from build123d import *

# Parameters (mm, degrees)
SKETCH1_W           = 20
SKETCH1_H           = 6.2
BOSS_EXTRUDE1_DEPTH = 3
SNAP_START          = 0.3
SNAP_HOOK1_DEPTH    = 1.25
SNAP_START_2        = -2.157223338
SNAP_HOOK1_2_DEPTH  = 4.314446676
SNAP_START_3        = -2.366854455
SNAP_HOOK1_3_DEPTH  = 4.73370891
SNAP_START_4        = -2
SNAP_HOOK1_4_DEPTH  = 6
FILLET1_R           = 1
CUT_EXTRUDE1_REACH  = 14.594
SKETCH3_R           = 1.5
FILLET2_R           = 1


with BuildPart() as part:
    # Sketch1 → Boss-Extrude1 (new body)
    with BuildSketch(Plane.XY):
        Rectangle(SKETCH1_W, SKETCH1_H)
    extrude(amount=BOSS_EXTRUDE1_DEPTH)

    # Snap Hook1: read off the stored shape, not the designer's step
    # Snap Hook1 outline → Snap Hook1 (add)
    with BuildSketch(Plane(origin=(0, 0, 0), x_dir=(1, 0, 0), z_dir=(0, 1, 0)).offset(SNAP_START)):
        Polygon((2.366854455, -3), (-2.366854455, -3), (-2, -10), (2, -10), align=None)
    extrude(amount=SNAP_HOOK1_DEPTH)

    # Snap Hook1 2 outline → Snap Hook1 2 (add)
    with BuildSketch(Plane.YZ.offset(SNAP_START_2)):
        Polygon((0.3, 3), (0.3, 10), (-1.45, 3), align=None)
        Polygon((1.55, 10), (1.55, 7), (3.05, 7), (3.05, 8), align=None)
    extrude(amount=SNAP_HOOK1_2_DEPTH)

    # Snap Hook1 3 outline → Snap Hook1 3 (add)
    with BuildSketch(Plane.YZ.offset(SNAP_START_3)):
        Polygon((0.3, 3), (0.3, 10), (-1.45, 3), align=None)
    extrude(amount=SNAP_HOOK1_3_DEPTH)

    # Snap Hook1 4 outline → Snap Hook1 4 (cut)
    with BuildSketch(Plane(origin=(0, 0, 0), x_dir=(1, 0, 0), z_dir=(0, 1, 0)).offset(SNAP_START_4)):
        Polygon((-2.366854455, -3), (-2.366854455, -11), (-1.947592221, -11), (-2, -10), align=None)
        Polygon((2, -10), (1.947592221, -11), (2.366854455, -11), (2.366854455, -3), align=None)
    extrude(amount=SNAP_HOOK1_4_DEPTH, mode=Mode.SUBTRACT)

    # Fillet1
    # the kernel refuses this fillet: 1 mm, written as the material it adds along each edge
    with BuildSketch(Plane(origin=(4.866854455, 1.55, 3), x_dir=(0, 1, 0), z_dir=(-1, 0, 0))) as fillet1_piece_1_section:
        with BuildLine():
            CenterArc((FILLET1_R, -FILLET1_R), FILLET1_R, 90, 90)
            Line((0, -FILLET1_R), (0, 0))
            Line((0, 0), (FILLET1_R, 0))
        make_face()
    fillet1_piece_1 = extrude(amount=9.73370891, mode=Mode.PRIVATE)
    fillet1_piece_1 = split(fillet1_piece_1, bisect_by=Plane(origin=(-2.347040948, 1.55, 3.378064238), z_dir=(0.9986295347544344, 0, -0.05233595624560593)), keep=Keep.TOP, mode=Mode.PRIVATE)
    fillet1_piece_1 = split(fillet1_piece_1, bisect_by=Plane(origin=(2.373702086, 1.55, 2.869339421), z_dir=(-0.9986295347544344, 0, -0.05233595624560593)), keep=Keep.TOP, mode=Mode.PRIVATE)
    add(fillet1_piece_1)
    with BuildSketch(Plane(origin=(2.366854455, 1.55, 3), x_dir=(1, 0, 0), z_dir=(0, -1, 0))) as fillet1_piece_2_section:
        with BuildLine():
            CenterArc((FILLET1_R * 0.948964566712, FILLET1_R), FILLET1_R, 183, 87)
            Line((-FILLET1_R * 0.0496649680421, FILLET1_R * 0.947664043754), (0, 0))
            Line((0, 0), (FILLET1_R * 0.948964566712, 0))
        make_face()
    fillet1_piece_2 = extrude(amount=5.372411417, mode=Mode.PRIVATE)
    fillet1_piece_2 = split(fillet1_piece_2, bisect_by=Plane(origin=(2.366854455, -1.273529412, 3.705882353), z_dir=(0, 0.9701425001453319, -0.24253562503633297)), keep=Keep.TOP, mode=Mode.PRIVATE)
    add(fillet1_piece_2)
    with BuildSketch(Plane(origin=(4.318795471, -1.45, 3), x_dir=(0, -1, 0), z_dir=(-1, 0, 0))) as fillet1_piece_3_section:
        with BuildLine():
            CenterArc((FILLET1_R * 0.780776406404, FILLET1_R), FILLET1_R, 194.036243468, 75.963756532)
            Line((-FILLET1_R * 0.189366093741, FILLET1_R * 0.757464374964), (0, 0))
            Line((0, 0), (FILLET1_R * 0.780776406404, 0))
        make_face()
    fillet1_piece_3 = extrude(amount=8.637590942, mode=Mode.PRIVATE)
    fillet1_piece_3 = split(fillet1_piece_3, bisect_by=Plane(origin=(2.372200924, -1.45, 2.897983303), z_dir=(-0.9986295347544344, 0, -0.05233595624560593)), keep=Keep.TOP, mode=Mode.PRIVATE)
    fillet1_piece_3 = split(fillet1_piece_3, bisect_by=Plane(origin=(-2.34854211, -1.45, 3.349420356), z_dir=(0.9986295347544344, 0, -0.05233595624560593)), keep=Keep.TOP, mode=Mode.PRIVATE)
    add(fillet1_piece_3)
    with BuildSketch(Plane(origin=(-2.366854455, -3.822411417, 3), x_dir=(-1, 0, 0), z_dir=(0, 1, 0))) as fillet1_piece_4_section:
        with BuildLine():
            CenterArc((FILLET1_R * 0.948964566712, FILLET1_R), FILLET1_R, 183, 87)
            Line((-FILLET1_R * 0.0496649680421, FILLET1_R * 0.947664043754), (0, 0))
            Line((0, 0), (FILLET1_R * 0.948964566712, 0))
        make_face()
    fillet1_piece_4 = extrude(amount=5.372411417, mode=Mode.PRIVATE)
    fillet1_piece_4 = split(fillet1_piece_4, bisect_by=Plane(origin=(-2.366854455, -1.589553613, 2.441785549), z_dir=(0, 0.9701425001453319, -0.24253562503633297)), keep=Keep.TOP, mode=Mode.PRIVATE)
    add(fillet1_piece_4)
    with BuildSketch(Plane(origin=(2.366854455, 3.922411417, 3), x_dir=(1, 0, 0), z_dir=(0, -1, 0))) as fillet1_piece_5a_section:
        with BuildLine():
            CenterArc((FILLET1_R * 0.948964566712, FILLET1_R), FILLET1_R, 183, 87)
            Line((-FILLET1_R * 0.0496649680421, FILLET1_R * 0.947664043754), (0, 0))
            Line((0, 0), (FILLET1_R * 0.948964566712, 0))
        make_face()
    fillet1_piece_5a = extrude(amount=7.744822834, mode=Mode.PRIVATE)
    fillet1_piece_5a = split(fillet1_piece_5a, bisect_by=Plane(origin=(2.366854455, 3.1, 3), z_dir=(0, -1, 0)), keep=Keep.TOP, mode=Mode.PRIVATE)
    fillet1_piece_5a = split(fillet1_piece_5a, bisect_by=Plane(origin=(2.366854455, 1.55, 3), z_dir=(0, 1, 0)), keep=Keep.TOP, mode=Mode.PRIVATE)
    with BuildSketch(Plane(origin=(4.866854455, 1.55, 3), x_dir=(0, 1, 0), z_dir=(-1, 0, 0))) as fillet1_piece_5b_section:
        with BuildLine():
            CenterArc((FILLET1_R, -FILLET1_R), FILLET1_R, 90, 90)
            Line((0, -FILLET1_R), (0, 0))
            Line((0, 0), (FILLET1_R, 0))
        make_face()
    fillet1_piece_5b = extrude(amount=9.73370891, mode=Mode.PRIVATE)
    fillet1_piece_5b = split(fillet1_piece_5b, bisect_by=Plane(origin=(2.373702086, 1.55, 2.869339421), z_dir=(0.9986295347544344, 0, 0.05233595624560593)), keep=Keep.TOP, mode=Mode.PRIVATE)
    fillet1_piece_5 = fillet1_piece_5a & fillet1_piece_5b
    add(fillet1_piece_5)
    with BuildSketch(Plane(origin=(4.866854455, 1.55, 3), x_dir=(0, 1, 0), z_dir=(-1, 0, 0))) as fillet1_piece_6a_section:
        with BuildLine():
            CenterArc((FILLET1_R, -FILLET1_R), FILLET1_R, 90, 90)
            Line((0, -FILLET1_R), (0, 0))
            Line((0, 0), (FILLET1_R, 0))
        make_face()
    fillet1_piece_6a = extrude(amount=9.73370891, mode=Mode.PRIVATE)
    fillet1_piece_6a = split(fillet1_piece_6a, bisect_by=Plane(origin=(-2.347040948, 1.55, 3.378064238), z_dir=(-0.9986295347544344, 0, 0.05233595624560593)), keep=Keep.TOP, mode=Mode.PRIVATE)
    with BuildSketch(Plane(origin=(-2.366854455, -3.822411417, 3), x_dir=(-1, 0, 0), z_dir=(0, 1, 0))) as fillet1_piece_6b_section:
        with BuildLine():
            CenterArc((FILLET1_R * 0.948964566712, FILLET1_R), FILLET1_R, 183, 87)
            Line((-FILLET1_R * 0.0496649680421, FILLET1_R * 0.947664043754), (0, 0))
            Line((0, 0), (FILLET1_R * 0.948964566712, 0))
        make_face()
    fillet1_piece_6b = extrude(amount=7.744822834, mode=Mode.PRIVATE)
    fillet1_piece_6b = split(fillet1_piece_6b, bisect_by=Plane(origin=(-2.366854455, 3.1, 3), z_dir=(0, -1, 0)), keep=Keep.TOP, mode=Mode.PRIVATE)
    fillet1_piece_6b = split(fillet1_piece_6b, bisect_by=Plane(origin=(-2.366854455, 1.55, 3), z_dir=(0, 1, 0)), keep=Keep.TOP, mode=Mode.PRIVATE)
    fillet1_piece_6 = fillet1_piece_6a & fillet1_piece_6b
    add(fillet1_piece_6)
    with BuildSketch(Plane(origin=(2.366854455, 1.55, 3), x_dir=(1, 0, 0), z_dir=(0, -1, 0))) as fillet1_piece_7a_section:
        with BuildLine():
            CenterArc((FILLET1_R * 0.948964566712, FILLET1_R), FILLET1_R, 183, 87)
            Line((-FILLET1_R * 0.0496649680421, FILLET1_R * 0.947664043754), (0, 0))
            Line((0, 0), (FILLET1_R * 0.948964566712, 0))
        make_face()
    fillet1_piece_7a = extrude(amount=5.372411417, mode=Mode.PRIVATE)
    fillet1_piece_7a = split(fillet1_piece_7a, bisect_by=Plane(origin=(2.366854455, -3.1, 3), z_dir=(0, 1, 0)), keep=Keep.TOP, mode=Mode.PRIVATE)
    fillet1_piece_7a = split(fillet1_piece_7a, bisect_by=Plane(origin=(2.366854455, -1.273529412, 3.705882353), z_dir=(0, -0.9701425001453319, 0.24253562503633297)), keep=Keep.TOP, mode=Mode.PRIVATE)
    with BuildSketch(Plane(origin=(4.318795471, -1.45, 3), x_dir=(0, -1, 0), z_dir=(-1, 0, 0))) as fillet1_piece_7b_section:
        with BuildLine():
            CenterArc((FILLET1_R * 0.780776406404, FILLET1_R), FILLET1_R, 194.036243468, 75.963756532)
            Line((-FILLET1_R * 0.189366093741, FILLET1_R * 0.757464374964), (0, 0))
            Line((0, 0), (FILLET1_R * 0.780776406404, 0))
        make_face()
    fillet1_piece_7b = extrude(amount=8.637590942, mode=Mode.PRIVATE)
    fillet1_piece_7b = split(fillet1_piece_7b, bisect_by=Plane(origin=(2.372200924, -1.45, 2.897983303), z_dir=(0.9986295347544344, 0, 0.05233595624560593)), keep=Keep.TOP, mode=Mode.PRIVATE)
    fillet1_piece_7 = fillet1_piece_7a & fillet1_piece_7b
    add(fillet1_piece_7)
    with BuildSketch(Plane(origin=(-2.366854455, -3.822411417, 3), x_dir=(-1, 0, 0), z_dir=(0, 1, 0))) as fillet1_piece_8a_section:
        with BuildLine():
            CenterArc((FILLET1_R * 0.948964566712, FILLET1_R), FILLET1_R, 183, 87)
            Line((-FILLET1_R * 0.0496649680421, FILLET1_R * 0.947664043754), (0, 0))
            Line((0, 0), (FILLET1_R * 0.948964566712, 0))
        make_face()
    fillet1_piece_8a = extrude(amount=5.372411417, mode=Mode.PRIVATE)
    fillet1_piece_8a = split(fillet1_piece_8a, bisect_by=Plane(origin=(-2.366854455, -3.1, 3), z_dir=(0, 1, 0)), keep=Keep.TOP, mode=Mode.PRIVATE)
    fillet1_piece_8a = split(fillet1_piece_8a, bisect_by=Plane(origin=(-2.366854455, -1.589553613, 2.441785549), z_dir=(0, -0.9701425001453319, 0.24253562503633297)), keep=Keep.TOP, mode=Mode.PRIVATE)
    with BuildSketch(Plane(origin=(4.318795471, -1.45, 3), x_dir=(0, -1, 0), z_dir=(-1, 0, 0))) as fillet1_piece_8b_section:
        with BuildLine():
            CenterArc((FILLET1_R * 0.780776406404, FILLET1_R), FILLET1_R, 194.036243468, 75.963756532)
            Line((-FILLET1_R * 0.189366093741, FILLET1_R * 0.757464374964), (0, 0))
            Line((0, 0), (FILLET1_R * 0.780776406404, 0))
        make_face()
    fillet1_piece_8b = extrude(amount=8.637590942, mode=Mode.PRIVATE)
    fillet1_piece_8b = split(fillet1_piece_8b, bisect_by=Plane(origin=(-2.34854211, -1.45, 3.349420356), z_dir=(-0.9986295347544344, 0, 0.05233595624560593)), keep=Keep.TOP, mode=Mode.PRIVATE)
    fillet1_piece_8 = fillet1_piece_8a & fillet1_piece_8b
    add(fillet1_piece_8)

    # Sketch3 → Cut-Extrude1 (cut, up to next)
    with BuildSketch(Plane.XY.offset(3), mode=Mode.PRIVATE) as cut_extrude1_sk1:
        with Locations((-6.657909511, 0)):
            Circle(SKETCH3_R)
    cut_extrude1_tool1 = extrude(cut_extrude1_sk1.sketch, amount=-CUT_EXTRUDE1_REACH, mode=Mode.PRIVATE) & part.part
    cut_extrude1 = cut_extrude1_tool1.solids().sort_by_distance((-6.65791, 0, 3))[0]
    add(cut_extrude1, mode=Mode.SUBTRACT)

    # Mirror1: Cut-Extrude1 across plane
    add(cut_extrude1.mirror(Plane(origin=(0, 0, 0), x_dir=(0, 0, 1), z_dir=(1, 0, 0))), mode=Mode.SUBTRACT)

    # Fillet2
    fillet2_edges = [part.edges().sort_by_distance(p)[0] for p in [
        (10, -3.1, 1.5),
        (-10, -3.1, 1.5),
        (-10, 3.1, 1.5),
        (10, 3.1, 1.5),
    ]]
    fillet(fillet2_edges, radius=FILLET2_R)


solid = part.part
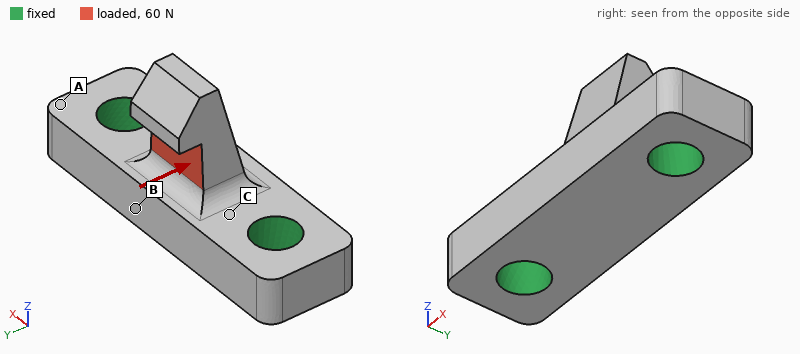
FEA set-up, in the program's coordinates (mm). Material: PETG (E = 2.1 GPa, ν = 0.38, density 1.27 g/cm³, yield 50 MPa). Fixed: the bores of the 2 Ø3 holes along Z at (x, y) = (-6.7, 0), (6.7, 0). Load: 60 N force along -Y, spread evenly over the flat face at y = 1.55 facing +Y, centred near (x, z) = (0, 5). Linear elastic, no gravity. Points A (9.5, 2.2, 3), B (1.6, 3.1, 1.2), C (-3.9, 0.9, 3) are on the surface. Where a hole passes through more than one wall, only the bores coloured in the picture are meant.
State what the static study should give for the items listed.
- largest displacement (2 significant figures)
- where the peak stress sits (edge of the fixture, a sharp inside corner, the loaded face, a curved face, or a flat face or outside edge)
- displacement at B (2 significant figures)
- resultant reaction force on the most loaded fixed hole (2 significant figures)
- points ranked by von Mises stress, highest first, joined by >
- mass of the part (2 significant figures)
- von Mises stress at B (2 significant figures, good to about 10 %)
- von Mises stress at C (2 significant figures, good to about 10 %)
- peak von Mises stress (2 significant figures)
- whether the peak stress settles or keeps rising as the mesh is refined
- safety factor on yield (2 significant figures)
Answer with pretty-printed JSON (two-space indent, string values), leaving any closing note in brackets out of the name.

{
  "largest displacement": "0.22 mm",
  "where the peak stress sits": "a curved face",
  "displacement at B": "0.039 mm",
  "resultant reaction force on the most loaded fixed hole": "30 N",
  "points ranked by von Mises stress, highest first, joined by >": "C > B > A",
  "mass of the part": "0.52 g",
  "von Mises stress at B": "7.3 MPa",
  "von Mises stress at C": "13 MPa",
  "peak von Mises stress": "40 MPa",
  "whether the peak stress settles or keeps rising as the mesh is refined": "settles",
  "safety factor on yield": "1.3"
}
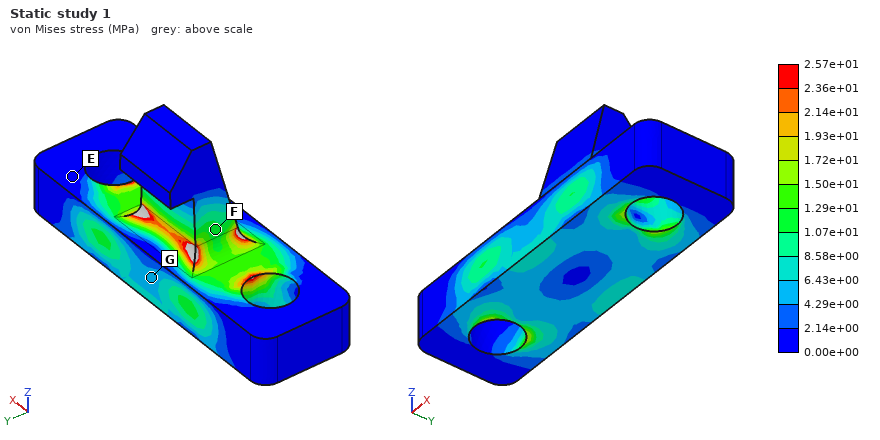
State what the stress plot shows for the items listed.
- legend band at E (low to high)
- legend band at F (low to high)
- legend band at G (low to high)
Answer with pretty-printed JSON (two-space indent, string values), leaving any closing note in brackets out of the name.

{
  "legend band at E": "0.00e+00 to 2.14e+00 MPa",
  "legend band at F": "1.07e+01 to 1.29e+01 MPa",
  "legend band at G": "4.29e+00 to 6.43e+00 MPa"
}
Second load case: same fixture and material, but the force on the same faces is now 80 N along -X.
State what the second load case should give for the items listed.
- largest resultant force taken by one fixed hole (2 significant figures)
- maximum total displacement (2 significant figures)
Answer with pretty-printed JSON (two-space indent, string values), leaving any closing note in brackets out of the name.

{
  "largest resultant force taken by one fixed hole": "54 N",
  "maximum total displacement": "0.13 mm"
}
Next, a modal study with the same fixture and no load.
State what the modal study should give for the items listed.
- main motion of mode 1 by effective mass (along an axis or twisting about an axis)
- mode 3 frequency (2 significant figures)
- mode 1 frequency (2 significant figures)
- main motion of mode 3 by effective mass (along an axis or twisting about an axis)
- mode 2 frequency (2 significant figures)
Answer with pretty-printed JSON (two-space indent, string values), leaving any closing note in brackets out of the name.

{
  "main motion of mode 1 by effective mass": "along Y",
  "mode 3 frequency": "18 kHz",
  "mode 1 frequency": "8000 Hz",
  "main motion of mode 3 by effective mass": "along Z",
  "mode 2 frequency": "13 kHz"
}
